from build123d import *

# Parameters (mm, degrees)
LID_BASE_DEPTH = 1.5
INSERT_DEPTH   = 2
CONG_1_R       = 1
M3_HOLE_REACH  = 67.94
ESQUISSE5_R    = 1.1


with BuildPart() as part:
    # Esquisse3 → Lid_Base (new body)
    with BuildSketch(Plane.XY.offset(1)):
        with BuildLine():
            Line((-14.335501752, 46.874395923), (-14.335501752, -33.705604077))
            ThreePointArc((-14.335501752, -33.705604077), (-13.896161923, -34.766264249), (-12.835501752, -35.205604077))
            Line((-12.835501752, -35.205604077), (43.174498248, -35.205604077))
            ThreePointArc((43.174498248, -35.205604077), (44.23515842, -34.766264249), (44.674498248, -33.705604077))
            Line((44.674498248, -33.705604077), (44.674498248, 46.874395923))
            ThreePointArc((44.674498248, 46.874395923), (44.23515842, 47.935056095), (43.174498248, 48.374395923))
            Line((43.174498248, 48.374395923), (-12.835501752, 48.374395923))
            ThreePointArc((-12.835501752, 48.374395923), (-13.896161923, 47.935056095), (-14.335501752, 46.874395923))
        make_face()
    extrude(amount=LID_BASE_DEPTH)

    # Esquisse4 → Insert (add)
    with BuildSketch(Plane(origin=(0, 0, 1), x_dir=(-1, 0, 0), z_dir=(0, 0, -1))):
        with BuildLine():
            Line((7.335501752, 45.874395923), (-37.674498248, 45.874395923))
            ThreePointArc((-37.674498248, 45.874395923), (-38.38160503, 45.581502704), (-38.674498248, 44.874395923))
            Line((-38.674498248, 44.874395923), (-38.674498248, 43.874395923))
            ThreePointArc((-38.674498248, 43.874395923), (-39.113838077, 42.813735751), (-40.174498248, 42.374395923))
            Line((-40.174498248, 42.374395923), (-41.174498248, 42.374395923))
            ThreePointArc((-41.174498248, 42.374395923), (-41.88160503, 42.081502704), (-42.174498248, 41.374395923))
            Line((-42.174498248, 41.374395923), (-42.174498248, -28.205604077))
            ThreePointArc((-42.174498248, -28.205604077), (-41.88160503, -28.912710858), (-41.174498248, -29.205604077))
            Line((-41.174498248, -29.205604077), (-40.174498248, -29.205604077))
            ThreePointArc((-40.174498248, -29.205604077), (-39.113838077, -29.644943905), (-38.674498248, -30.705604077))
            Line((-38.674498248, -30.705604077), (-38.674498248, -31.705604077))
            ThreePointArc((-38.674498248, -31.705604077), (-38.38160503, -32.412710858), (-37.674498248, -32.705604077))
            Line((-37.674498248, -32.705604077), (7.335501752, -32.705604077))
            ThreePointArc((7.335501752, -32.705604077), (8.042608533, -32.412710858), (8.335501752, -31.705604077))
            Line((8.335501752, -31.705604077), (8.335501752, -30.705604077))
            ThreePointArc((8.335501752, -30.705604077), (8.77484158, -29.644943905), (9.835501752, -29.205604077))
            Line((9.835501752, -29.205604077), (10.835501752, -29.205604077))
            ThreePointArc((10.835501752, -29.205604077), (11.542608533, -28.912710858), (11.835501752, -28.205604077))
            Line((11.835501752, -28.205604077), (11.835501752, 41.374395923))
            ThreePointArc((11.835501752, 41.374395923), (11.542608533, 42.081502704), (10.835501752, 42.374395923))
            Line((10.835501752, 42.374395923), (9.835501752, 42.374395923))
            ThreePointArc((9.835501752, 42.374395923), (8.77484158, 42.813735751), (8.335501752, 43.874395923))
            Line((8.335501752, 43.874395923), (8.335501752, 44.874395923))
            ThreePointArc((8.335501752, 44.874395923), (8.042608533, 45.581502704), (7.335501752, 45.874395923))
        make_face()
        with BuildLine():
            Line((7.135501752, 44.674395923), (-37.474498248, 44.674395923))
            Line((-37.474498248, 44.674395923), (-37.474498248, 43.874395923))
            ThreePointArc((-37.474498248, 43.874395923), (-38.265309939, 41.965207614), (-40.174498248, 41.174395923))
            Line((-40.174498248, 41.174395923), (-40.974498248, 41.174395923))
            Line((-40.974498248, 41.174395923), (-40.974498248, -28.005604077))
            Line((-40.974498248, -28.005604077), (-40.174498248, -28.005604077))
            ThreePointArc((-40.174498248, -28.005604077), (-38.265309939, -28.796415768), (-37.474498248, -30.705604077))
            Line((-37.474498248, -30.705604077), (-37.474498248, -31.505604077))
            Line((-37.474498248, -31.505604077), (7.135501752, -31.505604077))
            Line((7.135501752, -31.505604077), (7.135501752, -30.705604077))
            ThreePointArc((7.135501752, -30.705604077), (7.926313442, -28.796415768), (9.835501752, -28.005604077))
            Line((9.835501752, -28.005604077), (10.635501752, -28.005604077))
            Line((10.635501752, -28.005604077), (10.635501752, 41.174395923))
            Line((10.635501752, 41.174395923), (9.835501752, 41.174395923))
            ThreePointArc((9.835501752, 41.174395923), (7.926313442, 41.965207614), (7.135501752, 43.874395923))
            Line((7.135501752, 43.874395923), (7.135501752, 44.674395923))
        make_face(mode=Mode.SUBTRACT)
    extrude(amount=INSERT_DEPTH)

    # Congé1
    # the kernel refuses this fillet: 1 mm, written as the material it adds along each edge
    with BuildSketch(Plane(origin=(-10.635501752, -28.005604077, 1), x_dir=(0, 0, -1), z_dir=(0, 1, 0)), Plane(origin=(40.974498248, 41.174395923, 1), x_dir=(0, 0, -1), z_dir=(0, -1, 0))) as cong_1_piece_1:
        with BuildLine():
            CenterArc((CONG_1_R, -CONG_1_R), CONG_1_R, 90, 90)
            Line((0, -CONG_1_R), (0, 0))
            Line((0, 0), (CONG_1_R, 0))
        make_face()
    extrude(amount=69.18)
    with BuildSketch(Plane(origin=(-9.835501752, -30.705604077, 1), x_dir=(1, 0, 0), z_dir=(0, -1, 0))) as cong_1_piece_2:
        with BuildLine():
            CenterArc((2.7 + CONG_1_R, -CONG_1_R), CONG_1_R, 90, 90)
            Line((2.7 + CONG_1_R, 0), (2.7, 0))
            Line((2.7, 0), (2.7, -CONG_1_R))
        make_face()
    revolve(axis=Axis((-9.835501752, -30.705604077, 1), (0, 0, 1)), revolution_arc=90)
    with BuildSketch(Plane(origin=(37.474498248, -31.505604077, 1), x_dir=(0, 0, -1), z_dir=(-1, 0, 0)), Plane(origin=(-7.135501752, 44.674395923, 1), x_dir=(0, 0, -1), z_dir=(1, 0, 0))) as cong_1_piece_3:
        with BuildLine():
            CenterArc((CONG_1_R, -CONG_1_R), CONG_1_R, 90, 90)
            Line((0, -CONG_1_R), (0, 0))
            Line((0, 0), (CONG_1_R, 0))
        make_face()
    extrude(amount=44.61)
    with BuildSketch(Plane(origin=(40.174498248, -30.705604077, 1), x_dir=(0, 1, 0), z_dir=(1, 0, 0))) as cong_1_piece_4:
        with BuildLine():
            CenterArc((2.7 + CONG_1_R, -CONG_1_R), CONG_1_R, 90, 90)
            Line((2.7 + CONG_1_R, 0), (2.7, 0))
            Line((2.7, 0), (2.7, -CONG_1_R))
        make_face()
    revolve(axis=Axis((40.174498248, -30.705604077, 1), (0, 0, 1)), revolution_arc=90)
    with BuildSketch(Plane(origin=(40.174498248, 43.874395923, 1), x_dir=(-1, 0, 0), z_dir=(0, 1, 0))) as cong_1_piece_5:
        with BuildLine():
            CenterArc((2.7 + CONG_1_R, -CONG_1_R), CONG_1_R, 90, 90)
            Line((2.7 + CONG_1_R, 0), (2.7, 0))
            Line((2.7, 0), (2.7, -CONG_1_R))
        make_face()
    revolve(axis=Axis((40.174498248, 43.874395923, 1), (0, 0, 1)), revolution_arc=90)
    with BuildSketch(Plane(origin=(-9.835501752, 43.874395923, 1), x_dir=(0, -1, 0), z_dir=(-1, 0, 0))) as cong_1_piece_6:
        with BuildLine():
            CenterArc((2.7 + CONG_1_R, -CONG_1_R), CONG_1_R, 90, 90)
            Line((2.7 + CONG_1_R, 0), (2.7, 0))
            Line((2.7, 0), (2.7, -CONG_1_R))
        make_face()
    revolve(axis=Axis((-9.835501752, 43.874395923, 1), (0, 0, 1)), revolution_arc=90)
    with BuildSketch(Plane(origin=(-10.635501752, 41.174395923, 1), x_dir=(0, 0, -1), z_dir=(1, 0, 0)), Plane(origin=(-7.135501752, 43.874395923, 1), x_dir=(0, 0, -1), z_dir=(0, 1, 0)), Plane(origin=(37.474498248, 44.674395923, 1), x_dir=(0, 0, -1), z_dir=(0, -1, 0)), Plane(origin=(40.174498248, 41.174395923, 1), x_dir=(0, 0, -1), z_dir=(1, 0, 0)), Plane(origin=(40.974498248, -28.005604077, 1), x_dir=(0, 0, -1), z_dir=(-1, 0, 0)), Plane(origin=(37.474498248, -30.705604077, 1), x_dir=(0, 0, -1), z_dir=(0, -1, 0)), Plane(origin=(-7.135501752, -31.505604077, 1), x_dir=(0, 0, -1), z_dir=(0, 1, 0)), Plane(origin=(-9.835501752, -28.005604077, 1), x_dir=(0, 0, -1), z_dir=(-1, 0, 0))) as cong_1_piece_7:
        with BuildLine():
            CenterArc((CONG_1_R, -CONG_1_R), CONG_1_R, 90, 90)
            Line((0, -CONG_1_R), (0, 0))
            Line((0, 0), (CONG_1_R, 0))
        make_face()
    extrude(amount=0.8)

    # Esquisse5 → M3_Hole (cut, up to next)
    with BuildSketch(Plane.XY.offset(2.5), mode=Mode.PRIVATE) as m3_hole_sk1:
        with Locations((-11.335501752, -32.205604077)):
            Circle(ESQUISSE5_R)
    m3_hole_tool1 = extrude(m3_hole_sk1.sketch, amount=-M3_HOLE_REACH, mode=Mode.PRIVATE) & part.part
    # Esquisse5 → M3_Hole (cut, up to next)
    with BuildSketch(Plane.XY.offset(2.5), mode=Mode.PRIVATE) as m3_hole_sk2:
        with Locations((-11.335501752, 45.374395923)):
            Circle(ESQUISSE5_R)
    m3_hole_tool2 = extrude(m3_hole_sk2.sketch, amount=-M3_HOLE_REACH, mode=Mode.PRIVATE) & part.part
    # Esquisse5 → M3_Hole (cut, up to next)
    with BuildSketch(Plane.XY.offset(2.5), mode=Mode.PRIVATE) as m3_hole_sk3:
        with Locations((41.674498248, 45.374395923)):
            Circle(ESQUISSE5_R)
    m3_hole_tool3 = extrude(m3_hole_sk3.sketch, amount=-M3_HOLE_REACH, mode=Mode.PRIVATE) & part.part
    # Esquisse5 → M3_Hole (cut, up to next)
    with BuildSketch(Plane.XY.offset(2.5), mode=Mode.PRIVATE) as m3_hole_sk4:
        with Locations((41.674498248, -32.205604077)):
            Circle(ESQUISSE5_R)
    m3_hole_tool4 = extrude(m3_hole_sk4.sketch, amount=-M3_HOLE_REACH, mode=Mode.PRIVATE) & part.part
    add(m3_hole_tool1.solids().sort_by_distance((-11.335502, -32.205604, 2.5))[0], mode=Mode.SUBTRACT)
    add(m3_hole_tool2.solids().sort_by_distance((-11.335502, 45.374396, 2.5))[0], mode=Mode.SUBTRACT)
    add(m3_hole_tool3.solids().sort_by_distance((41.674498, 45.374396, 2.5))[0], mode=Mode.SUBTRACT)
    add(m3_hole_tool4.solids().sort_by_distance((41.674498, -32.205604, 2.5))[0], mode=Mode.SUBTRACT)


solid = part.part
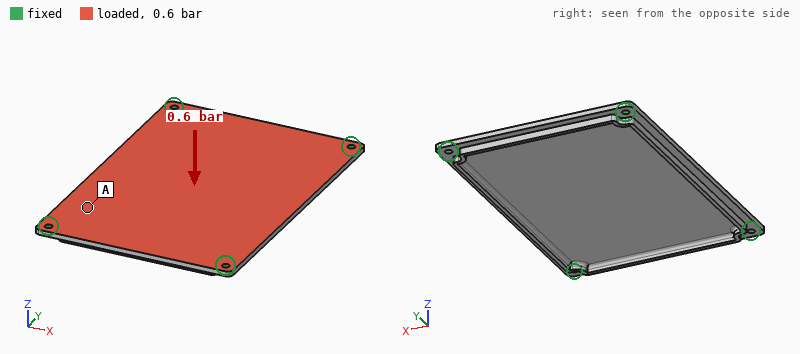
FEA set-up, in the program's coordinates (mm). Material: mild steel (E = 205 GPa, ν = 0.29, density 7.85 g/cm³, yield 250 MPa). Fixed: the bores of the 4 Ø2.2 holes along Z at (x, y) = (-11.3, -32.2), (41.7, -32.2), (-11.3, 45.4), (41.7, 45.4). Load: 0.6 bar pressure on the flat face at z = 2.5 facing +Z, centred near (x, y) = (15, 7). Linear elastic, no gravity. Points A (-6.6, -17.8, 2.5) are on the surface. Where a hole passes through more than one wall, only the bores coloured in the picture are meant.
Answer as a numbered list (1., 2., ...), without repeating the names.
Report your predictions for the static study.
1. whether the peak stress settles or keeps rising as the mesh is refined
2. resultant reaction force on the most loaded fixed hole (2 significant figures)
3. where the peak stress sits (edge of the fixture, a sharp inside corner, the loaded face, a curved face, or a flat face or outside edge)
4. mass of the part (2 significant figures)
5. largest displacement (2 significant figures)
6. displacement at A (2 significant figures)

1. keeps rising
2. 82 N
3. edge of the fixture
4. 63 g
5. 0.12 mm
6. 0.049 mm
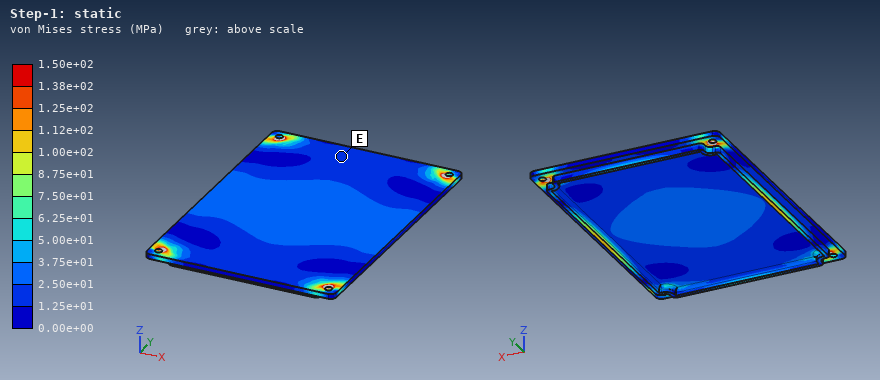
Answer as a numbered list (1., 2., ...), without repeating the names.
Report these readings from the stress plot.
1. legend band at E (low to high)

1. 1.25e+01 to 2.50e+01 MPa
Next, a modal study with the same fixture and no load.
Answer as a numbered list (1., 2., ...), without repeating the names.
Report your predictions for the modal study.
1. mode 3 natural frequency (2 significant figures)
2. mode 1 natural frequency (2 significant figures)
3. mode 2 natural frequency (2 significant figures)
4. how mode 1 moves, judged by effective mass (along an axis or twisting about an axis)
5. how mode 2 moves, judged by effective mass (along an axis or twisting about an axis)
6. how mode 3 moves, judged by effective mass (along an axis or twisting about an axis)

1. 2800 Hz
2. 1200 Hz
3. 2000 Hz
4. along Z
5. twisting about Y
6. twisting about X
